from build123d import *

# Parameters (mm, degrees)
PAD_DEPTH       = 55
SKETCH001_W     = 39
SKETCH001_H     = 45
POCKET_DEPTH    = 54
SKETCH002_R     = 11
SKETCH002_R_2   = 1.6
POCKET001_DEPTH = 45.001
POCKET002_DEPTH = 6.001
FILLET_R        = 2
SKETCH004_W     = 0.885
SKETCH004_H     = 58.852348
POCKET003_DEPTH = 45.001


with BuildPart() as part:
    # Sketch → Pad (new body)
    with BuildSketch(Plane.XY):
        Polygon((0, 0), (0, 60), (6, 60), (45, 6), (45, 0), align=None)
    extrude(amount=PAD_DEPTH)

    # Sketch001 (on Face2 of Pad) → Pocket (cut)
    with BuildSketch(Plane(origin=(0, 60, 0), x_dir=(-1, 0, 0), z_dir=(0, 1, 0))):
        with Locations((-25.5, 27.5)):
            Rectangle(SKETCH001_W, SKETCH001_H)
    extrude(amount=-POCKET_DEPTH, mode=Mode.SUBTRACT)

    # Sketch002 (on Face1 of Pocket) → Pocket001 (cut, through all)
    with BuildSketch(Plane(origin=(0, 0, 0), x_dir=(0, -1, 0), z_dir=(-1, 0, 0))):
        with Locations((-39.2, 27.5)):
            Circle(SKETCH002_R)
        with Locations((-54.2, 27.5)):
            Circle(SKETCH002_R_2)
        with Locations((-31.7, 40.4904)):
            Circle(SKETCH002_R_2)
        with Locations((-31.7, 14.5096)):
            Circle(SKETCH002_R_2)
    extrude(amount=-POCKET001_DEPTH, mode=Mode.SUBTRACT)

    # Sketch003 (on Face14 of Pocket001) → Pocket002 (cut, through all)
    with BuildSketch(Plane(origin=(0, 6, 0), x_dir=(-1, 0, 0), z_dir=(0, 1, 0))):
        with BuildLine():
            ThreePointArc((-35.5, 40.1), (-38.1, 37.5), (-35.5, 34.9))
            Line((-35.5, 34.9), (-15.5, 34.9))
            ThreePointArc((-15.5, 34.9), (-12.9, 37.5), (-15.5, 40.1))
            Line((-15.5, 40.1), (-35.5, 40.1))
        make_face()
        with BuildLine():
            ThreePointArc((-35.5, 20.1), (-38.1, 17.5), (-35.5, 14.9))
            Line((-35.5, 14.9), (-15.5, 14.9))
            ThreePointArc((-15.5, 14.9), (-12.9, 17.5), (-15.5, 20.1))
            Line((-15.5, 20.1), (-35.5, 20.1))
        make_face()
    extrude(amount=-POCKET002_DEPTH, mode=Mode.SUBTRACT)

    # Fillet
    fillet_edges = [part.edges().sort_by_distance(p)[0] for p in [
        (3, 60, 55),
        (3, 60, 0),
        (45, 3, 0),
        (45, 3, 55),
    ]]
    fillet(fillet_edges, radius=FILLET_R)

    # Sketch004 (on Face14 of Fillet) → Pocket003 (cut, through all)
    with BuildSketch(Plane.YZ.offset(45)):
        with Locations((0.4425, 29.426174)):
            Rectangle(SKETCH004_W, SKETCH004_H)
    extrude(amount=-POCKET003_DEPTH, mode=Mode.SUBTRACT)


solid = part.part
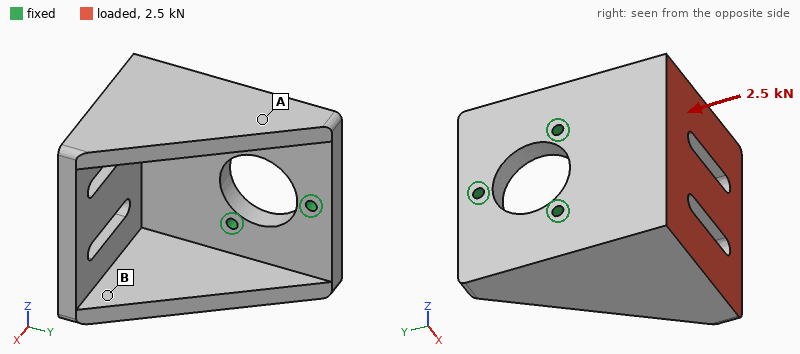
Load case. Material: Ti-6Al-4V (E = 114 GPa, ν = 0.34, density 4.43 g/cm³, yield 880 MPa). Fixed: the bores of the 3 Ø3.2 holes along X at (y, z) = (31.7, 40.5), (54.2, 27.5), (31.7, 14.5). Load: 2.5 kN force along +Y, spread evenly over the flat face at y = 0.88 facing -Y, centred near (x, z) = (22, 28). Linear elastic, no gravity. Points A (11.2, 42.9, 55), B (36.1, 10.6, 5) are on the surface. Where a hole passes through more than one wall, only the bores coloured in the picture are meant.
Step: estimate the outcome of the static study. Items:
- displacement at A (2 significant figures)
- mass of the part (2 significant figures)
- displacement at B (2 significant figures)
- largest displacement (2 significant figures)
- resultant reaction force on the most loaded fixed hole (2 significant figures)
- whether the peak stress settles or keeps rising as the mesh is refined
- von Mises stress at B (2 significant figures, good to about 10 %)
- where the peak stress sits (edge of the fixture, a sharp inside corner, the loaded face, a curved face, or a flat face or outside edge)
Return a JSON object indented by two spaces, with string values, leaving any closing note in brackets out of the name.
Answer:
{
  "displacement at A": "0.040 mm",
  "mass of the part": "170 g",
  "displacement at B": "0.10 mm",
  "largest displacement": "0.17 mm",
  "resultant reaction force on the most loaded fixed hole": "1.3 kN",
  "whether the peak stress settles or keeps rising as the mesh is refined": "keeps rising",
  "von Mises stress at B": "30 MPa",
  "where the peak stress sits": "edge of the fixture"
}
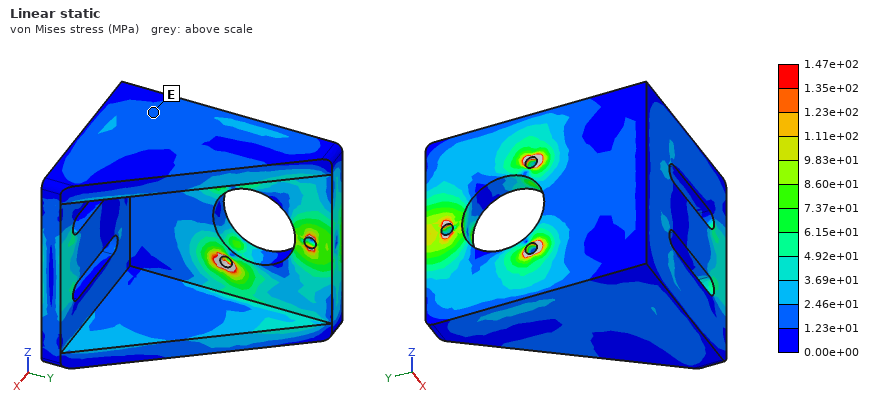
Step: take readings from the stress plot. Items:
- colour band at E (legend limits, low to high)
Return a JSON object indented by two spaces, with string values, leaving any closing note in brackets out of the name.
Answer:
{
  "colour band at E": "1.23e+01 to 2.46e+01 MPa"
}
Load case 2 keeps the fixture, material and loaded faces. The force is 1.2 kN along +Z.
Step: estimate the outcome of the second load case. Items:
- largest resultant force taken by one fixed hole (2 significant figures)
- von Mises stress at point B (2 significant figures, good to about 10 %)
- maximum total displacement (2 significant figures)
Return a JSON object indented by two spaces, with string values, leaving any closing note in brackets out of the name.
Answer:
{
  "largest resultant force taken by one fixed hole": "1.4 kN",
  "von Mises stress at point B": "13 MPa",
  "maximum total displacement": "65 µm"
}
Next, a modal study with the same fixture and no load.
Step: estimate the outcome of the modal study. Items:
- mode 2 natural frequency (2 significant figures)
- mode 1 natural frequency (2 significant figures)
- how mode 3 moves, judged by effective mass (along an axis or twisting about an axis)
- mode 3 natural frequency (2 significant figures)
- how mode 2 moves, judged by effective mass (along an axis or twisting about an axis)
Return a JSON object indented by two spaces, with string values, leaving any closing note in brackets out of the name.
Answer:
{
  "mode 2 natural frequency": "2500 Hz",
  "mode 1 natural frequency": "2200 Hz",
  "how mode 3 moves, judged by effective mass": "along X",
  "mode 3 natural frequency": "5600 Hz",
  "how mode 2 moves, judged by effective mass": "along Z"
}
